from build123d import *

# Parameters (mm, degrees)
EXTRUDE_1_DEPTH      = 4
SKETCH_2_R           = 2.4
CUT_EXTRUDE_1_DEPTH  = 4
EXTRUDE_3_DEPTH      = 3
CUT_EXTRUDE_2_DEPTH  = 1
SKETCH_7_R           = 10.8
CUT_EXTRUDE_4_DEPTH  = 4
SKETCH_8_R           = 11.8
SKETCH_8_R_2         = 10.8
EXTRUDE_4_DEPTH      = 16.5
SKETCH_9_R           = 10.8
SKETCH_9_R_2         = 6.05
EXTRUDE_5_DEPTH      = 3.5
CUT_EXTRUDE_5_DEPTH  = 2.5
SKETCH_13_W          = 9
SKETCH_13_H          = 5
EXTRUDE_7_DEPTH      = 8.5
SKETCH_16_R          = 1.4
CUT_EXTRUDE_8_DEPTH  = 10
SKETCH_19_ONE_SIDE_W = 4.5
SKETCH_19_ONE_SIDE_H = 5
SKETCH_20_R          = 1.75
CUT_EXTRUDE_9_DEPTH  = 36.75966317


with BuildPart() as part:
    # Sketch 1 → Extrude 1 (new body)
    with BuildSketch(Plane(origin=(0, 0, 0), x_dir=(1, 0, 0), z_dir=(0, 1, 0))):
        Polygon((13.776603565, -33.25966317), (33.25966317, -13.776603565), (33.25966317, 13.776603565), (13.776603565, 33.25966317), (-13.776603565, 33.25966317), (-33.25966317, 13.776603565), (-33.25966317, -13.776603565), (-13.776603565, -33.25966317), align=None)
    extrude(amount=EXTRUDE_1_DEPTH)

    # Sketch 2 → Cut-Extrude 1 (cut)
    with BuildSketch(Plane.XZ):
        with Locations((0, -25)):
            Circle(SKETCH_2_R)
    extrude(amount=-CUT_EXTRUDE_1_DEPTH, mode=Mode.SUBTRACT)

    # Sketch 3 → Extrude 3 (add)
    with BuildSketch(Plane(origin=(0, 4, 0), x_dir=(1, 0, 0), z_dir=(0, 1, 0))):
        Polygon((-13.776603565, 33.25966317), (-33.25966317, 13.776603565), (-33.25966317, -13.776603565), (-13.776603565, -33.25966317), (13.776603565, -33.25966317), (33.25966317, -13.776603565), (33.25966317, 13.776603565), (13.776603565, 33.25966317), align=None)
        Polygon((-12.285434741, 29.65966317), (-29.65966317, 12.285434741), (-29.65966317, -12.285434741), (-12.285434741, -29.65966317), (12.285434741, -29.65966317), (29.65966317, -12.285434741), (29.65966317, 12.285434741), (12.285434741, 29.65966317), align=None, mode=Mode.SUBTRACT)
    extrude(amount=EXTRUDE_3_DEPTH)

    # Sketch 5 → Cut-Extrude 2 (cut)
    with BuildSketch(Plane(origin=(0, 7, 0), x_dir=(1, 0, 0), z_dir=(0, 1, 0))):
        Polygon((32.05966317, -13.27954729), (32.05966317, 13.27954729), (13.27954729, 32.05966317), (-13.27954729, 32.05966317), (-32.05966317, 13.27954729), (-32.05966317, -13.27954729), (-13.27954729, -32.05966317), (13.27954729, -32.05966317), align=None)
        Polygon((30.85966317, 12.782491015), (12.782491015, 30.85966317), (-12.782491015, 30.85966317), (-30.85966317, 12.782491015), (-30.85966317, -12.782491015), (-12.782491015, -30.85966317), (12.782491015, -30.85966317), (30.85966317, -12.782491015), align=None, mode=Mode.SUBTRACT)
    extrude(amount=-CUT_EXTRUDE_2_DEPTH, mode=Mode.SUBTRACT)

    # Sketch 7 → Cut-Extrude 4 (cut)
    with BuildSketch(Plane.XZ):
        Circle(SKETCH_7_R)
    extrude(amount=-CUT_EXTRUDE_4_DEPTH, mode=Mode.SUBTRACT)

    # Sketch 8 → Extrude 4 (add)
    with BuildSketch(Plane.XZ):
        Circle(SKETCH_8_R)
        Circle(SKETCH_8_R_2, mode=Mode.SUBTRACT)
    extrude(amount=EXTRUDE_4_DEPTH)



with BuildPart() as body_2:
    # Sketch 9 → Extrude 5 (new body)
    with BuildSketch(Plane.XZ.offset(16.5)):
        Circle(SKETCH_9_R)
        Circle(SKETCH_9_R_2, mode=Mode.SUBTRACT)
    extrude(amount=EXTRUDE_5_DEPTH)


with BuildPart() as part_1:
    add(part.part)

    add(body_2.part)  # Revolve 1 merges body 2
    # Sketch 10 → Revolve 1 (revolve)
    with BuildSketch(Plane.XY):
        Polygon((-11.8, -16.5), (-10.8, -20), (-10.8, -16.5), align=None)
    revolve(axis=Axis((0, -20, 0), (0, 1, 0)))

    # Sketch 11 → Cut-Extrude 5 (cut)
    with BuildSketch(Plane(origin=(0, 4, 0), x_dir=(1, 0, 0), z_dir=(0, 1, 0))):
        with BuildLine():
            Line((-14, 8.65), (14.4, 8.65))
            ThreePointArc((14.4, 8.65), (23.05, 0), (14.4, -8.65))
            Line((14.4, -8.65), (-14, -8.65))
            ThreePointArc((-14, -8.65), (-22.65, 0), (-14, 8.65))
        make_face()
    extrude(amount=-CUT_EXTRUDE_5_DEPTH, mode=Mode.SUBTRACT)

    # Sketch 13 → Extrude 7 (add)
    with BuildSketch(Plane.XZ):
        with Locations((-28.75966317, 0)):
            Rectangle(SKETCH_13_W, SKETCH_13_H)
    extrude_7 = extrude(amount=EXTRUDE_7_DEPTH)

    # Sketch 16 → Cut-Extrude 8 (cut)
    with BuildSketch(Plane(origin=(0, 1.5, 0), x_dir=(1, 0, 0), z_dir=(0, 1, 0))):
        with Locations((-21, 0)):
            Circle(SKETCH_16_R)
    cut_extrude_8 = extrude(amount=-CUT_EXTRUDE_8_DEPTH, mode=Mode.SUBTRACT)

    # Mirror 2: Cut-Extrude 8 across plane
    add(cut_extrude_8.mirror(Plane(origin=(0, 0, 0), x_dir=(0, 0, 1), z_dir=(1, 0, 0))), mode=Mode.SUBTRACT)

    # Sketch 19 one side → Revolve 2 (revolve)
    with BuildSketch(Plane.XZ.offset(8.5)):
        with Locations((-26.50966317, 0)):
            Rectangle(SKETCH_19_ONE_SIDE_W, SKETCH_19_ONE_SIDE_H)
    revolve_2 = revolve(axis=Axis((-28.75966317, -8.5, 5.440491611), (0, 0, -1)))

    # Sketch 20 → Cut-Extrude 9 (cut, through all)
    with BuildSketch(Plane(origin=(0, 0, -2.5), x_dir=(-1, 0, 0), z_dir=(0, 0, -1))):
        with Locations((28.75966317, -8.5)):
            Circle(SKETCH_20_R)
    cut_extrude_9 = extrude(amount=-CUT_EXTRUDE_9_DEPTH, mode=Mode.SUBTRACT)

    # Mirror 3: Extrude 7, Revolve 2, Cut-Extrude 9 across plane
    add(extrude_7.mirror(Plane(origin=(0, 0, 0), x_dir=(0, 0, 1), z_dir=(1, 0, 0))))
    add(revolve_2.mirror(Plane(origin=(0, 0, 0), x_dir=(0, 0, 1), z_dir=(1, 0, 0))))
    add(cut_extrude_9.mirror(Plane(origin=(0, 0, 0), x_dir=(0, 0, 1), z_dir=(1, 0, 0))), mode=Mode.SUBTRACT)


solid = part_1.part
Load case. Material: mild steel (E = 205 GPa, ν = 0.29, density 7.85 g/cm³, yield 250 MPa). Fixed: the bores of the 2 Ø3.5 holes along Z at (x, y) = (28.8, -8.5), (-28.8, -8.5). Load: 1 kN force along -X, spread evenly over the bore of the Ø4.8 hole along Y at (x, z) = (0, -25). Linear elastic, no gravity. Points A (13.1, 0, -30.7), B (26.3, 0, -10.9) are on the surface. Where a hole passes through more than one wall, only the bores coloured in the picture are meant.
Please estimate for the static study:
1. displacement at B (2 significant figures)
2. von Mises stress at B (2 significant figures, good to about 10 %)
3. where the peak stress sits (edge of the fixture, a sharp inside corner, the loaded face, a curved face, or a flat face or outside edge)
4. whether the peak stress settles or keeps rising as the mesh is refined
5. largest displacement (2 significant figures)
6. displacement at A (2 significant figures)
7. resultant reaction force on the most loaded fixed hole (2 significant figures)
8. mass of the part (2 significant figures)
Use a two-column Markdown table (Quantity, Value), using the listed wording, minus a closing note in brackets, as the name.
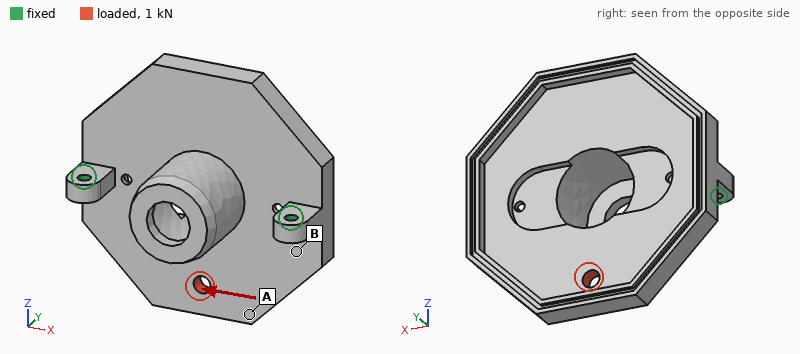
| Quantity | Value |
|---|---|
| displacement at B | 9.1 µm |
| von Mises stress at B | 21 MPa |
| where the peak stress sits | edge of the fixture |
| whether the peak stress settles or keeps rising as the mesh is refined | keeps rising |
| largest displacement | 14 µm |
| displacement at A | 13 µm |
| resultant reaction force on the most loaded fixed hole | 660 N |
| mass of the part | 140 g |
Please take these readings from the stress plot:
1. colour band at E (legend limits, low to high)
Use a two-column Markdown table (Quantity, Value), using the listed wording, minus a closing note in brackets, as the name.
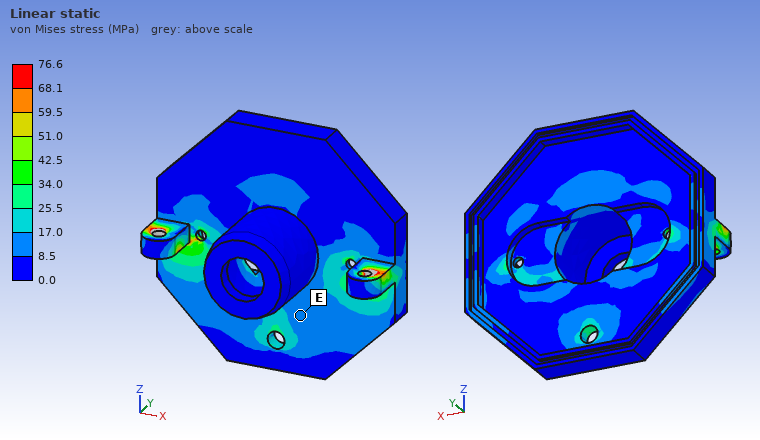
| Quantity | Value |
|---|---|
| colour band at E | 8.5 to 17.0 MPa |
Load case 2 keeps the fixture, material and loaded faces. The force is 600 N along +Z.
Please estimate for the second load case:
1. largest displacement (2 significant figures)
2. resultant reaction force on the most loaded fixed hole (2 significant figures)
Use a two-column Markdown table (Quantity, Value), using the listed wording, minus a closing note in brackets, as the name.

| Quantity | Value |
|---|---|
| largest displacement | 30 µm |
| resultant reaction force on the most loaded fixed hole | 300 N |
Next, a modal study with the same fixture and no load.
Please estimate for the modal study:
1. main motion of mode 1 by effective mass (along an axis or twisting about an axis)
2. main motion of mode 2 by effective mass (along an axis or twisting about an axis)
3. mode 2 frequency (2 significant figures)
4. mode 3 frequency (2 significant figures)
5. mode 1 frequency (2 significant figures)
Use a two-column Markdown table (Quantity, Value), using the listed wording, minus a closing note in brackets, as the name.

| Quantity | Value |
|---|---|
| main motion of mode 1 by effective mass | twisting about X |
| main motion of mode 2 by effective mass | along Y |
| mode 2 frequency | 2800 Hz |
| mode 3 frequency | 4700 Hz |
| mode 1 frequency | 1300 Hz |
